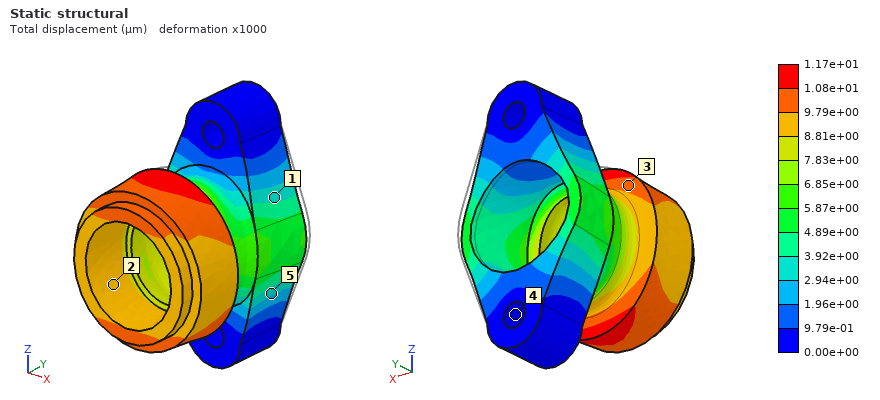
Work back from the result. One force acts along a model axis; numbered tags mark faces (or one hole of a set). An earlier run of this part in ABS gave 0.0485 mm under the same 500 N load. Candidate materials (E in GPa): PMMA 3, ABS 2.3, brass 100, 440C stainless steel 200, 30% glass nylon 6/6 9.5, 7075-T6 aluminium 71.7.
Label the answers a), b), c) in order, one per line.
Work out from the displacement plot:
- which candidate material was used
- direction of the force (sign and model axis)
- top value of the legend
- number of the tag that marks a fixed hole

a) 30% glass nylon 6/6
b) -Y
c) 1.17e+01 µm
d) 4
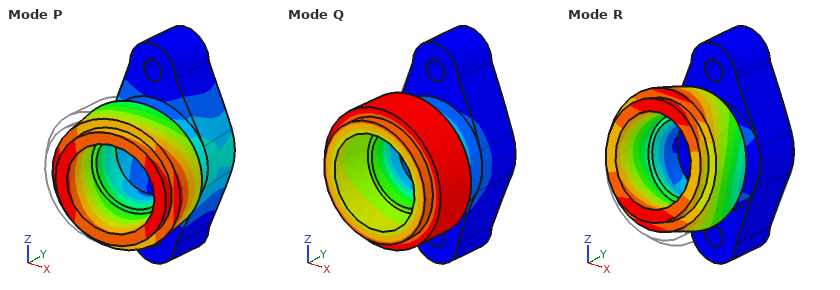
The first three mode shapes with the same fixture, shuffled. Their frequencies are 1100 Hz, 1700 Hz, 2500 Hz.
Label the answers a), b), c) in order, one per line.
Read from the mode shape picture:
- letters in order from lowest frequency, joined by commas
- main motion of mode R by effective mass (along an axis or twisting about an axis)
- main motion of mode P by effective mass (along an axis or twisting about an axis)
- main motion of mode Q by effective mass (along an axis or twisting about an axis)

a) P, R, Q
b) along Z
c) along X
d) twisting about Y
